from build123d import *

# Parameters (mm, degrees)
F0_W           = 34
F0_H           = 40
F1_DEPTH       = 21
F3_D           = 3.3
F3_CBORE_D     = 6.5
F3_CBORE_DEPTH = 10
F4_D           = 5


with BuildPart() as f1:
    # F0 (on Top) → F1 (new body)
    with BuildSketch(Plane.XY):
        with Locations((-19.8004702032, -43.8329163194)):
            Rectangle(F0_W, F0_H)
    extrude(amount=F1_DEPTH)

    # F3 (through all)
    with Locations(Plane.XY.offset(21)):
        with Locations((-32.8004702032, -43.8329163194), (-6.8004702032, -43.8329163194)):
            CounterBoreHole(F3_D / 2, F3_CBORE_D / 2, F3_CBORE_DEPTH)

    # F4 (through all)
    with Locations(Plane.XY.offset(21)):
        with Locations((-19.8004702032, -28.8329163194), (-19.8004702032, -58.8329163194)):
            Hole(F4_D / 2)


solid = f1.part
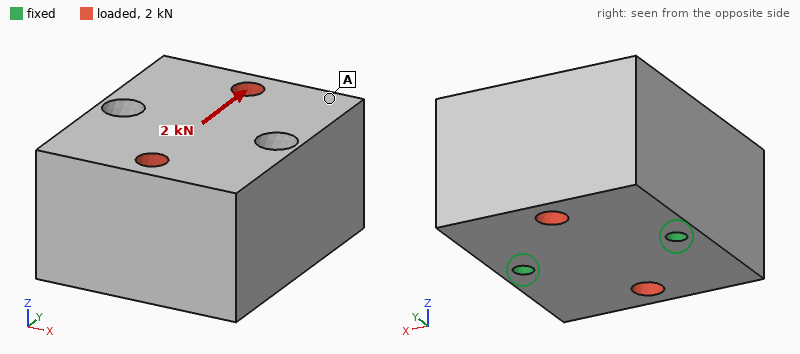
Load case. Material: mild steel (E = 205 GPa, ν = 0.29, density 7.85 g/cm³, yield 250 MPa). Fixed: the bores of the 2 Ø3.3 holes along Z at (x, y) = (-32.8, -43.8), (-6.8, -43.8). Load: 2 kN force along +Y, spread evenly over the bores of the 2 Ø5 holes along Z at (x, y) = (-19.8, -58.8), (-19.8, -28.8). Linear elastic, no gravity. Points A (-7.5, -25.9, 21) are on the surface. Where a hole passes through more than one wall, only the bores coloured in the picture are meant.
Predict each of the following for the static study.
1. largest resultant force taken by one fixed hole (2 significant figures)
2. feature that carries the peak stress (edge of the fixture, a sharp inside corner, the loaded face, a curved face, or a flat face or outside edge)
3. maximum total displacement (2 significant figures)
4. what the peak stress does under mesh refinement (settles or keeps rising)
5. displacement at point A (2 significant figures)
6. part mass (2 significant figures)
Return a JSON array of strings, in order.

["1.0 kN", "edge of the fixture", "2.1 µm", "keeps rising", "1.7 µm", "210 g"]
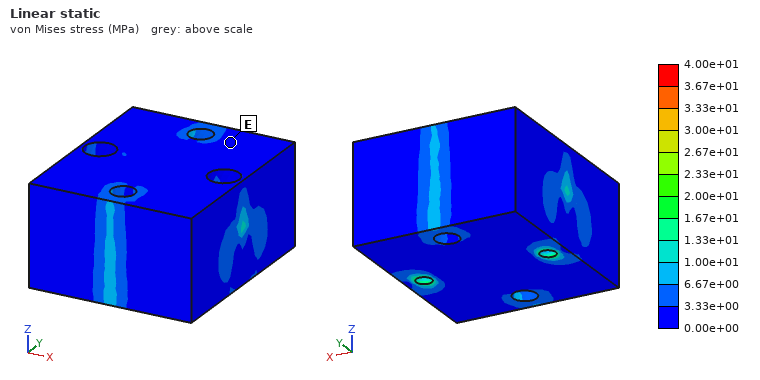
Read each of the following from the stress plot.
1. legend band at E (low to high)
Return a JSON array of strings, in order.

["0.00e+00 to 3.33e+00 MPa"]
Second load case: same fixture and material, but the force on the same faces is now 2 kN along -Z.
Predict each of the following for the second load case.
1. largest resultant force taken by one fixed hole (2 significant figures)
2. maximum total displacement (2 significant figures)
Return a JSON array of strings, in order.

["1.0 kN", "1.3 µm"]
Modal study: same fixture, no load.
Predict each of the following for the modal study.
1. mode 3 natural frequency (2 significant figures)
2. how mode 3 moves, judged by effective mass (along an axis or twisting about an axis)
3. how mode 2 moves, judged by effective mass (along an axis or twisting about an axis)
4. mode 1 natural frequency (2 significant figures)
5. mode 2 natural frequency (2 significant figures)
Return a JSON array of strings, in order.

["22 kHz", "along X", "along Z", "9500 Hz", "21 kHz"]
